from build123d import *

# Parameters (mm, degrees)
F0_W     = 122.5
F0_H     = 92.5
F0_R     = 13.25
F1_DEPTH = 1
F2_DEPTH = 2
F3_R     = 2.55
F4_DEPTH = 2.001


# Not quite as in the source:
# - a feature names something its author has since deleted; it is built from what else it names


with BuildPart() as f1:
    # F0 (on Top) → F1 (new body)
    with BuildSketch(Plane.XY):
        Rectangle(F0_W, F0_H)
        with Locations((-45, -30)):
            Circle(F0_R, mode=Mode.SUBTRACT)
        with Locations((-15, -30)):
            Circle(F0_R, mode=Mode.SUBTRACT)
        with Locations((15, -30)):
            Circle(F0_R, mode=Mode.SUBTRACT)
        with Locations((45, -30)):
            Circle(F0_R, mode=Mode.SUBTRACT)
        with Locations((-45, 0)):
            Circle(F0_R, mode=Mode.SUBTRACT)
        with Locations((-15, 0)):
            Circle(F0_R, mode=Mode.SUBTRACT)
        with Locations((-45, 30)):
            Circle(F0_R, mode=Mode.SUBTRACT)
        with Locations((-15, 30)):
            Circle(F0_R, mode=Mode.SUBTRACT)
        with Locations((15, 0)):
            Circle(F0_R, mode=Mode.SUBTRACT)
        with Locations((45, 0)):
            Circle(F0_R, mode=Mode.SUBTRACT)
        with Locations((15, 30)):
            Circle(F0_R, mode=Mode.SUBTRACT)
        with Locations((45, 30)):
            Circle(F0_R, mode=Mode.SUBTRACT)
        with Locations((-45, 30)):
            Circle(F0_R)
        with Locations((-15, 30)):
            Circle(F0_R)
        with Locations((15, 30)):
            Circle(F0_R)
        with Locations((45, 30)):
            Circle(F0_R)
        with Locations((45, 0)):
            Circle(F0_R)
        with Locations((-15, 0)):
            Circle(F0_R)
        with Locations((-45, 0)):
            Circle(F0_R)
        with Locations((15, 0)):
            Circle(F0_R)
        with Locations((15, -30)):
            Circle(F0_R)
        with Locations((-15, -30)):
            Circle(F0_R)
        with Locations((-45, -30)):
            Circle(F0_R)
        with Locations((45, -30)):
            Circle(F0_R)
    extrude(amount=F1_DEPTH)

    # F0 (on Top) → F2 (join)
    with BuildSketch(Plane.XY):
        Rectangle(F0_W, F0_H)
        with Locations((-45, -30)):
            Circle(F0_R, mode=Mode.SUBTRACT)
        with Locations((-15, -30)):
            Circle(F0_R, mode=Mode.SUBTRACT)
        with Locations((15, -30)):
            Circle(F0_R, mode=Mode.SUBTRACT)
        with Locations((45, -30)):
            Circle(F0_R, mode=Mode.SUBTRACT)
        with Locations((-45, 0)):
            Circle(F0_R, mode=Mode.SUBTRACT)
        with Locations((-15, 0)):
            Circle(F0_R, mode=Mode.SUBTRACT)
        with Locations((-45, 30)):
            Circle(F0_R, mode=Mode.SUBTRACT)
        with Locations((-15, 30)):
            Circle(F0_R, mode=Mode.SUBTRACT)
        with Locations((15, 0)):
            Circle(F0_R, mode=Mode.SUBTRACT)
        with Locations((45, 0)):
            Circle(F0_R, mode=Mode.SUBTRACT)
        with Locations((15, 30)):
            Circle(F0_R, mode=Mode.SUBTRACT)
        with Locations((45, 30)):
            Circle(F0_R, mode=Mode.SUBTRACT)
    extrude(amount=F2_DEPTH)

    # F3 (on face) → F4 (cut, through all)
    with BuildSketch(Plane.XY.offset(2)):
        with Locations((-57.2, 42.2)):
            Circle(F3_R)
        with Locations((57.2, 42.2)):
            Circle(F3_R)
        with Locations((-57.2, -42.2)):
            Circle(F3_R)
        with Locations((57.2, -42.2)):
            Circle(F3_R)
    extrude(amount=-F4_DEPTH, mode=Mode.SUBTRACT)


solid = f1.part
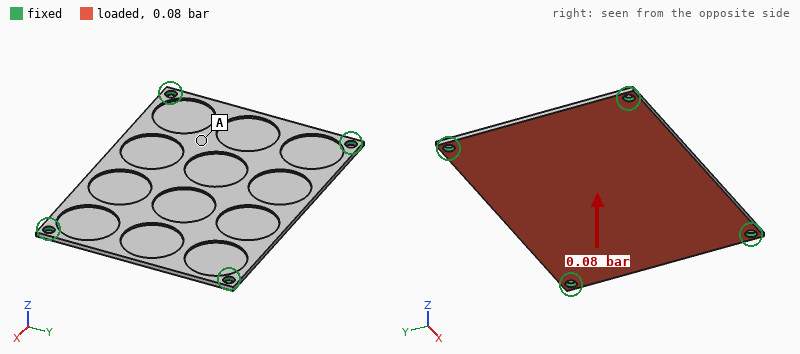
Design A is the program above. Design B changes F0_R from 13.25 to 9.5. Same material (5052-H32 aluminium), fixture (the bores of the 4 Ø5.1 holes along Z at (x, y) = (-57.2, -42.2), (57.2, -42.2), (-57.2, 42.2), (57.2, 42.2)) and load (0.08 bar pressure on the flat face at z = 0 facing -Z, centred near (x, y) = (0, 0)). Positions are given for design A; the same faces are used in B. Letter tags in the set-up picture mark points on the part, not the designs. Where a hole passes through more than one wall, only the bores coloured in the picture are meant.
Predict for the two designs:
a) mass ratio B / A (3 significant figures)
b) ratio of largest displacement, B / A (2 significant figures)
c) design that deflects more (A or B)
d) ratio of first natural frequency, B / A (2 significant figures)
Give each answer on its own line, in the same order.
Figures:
1.20
0.58
A
1.2
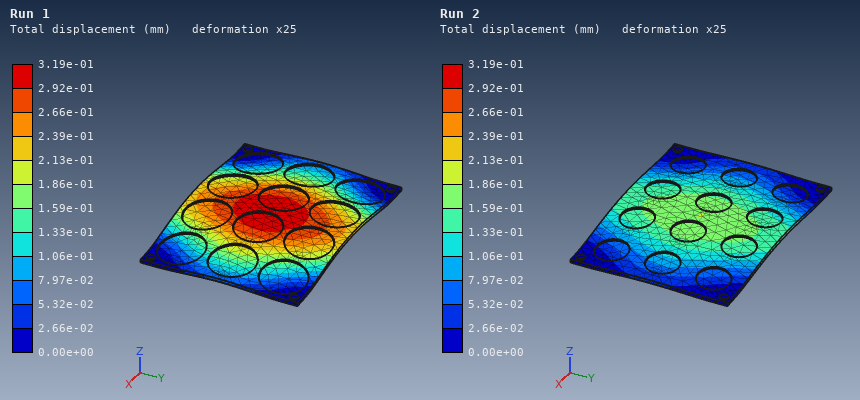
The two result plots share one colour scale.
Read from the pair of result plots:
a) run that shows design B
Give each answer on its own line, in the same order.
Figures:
Run 2
